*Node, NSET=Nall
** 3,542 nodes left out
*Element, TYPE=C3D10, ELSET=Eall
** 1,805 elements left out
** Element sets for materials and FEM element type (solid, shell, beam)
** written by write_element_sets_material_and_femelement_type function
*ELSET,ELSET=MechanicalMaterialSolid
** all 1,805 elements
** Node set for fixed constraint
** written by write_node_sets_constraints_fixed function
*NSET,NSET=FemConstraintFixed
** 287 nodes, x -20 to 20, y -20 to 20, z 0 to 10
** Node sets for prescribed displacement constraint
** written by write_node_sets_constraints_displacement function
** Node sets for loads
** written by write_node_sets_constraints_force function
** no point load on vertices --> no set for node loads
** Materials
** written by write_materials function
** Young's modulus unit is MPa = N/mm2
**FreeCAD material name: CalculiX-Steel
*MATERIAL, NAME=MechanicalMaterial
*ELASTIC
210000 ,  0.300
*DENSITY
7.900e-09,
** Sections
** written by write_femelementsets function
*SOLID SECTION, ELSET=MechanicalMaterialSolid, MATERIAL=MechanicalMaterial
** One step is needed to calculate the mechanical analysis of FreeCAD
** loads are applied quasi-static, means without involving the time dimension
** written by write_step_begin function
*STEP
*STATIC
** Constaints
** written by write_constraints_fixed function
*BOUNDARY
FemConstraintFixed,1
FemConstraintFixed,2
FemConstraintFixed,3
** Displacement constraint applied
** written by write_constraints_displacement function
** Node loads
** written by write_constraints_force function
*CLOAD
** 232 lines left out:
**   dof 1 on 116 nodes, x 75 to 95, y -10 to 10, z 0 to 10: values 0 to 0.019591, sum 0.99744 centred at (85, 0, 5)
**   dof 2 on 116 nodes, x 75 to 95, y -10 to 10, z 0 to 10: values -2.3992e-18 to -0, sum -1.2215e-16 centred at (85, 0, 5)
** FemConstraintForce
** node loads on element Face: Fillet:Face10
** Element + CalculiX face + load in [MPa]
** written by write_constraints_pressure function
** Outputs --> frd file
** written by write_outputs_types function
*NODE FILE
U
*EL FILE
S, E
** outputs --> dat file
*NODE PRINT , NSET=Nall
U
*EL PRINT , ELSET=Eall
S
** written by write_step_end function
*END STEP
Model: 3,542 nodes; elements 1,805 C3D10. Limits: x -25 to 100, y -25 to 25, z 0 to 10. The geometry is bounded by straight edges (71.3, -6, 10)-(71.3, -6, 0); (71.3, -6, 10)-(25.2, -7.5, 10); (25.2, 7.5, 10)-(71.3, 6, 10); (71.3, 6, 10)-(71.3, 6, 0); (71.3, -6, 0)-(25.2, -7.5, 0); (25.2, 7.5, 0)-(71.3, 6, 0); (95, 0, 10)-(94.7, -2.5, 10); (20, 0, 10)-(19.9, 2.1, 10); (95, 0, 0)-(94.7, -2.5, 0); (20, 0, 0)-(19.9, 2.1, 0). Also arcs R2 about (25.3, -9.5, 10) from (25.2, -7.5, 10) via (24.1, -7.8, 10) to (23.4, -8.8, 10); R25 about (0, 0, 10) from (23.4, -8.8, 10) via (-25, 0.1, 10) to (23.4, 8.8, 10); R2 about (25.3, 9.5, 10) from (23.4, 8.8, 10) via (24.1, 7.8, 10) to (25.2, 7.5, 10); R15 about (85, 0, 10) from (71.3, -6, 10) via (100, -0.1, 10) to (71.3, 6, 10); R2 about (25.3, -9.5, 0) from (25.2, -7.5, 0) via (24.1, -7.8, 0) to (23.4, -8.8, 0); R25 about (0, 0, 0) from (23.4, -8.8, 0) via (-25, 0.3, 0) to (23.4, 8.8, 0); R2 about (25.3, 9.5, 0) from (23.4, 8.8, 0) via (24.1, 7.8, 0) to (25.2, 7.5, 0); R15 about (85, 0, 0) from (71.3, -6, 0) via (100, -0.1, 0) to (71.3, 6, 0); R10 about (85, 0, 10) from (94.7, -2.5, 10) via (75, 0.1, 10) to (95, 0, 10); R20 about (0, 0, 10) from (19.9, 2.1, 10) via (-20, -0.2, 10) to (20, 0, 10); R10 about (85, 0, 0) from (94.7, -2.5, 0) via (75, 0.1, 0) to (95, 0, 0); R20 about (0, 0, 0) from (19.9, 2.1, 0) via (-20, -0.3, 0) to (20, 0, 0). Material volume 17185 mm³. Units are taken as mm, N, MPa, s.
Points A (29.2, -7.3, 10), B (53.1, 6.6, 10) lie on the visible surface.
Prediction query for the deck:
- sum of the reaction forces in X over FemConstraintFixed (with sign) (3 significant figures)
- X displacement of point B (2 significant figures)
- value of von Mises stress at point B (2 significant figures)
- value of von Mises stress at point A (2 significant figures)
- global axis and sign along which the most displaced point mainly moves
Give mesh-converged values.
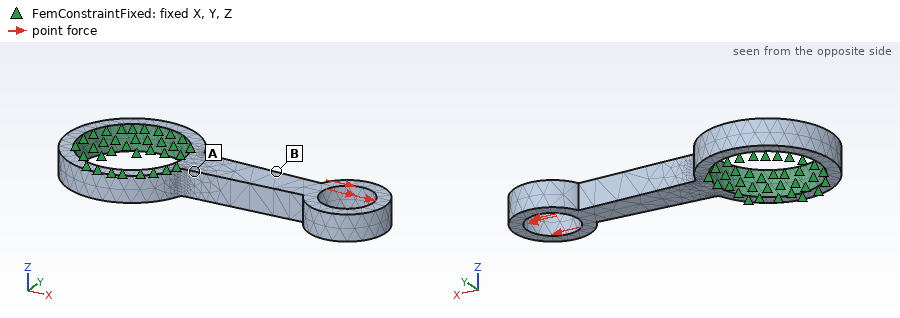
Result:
-0.997 N
1.1e-06 mm
0.0075 MPa
0.0066 MPa
+X
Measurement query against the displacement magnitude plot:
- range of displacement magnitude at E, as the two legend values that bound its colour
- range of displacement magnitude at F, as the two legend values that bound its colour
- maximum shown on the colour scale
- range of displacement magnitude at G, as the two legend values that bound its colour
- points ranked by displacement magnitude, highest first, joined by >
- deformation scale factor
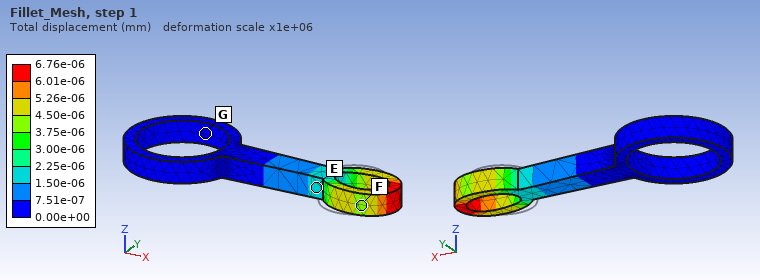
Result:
1.50e-06 to 2.25e-06 mm
3.75e-06 to 4.50e-06 mm
6.76e-06 mm
0.00e+00 to 7.51e-07 mm
F > E > G
1e+06
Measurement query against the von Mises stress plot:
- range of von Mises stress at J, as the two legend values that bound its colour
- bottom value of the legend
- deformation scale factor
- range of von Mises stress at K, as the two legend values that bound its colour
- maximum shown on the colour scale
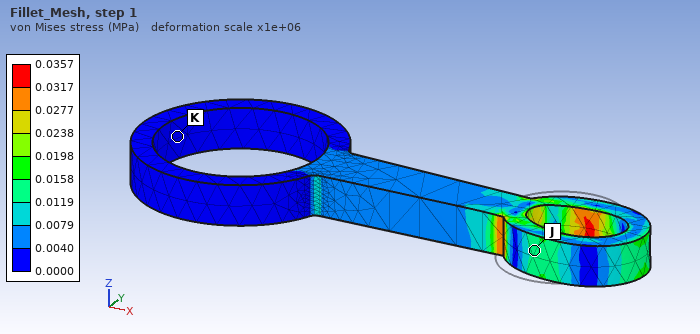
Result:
0.0119 to 0.0158 MPa
0.0000 MPa
1e+06
0.0000 to 0.0040 MPa
0.0357 MPa
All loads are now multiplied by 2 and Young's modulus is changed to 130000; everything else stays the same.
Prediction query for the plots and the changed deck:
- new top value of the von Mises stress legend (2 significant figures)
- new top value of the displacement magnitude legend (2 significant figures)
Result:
0.071 MPa
2.2e-05 mm
